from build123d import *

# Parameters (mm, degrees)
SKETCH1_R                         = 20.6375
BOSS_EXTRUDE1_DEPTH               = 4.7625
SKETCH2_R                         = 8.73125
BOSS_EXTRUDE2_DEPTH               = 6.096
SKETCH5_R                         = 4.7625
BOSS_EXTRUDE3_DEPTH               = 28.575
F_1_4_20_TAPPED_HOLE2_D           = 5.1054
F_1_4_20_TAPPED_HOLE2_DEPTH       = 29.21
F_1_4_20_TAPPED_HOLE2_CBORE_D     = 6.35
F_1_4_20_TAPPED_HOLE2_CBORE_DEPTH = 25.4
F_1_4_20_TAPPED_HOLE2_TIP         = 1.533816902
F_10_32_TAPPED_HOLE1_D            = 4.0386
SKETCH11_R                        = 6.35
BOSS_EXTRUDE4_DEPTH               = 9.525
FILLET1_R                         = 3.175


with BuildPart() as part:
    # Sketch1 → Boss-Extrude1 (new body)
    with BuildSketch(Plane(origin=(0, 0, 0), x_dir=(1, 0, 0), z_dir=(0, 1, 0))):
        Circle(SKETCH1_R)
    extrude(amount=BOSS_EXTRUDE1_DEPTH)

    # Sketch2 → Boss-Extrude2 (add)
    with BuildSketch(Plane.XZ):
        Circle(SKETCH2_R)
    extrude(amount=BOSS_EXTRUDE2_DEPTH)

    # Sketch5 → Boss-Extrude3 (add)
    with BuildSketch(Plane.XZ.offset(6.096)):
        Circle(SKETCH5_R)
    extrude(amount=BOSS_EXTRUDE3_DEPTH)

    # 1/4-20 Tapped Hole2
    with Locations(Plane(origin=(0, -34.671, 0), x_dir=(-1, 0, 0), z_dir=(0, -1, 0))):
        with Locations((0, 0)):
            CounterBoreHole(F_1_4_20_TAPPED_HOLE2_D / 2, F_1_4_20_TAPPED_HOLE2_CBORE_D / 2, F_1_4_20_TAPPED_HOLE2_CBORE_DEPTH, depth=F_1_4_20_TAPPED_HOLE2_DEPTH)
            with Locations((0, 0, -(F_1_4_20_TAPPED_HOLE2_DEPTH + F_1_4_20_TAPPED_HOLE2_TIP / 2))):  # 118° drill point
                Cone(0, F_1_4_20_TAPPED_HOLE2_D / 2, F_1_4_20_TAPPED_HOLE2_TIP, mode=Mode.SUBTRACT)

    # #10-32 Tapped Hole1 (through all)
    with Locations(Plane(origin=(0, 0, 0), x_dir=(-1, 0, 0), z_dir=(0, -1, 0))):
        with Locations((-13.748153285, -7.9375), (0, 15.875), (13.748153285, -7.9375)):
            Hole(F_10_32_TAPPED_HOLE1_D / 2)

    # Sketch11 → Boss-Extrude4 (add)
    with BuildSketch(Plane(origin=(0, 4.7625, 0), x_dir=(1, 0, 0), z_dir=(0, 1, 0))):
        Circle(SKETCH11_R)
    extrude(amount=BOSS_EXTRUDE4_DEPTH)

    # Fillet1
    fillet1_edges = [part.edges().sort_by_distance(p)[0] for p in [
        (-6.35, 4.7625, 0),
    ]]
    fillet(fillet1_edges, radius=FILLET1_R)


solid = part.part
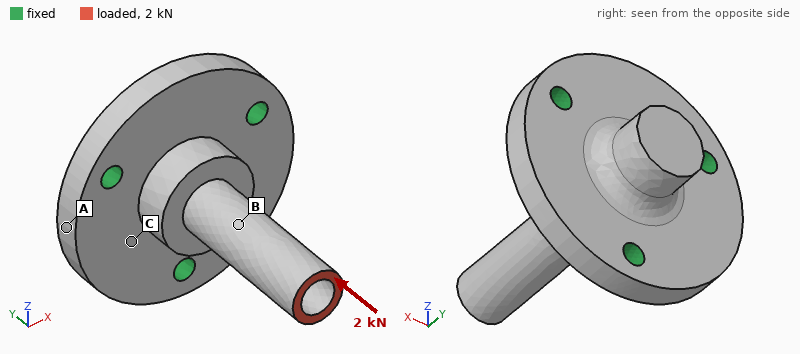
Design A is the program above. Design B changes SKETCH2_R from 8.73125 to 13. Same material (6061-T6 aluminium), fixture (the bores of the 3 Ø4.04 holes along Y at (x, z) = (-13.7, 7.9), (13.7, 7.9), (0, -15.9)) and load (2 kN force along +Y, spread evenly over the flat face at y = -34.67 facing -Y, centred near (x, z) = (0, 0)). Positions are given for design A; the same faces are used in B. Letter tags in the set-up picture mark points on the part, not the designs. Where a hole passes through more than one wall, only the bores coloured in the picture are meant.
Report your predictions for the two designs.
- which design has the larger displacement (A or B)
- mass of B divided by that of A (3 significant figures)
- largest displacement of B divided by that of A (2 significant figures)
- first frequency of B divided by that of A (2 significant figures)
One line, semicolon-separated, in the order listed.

A; 1.18; 0.89; 1.1
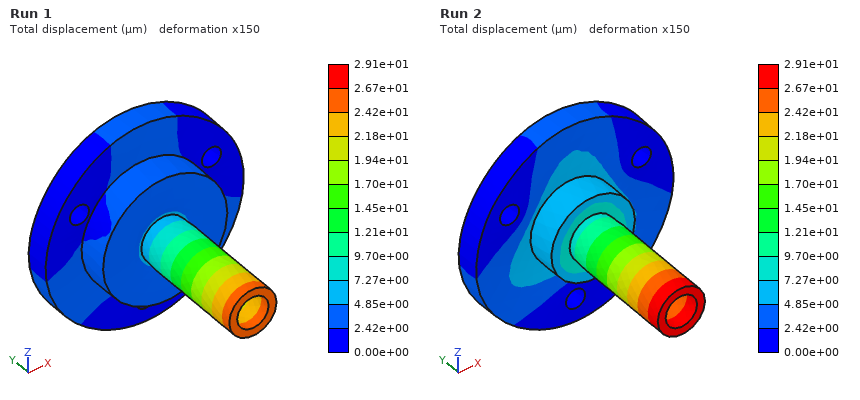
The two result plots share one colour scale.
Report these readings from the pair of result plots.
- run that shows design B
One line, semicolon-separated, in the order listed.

Run 1
